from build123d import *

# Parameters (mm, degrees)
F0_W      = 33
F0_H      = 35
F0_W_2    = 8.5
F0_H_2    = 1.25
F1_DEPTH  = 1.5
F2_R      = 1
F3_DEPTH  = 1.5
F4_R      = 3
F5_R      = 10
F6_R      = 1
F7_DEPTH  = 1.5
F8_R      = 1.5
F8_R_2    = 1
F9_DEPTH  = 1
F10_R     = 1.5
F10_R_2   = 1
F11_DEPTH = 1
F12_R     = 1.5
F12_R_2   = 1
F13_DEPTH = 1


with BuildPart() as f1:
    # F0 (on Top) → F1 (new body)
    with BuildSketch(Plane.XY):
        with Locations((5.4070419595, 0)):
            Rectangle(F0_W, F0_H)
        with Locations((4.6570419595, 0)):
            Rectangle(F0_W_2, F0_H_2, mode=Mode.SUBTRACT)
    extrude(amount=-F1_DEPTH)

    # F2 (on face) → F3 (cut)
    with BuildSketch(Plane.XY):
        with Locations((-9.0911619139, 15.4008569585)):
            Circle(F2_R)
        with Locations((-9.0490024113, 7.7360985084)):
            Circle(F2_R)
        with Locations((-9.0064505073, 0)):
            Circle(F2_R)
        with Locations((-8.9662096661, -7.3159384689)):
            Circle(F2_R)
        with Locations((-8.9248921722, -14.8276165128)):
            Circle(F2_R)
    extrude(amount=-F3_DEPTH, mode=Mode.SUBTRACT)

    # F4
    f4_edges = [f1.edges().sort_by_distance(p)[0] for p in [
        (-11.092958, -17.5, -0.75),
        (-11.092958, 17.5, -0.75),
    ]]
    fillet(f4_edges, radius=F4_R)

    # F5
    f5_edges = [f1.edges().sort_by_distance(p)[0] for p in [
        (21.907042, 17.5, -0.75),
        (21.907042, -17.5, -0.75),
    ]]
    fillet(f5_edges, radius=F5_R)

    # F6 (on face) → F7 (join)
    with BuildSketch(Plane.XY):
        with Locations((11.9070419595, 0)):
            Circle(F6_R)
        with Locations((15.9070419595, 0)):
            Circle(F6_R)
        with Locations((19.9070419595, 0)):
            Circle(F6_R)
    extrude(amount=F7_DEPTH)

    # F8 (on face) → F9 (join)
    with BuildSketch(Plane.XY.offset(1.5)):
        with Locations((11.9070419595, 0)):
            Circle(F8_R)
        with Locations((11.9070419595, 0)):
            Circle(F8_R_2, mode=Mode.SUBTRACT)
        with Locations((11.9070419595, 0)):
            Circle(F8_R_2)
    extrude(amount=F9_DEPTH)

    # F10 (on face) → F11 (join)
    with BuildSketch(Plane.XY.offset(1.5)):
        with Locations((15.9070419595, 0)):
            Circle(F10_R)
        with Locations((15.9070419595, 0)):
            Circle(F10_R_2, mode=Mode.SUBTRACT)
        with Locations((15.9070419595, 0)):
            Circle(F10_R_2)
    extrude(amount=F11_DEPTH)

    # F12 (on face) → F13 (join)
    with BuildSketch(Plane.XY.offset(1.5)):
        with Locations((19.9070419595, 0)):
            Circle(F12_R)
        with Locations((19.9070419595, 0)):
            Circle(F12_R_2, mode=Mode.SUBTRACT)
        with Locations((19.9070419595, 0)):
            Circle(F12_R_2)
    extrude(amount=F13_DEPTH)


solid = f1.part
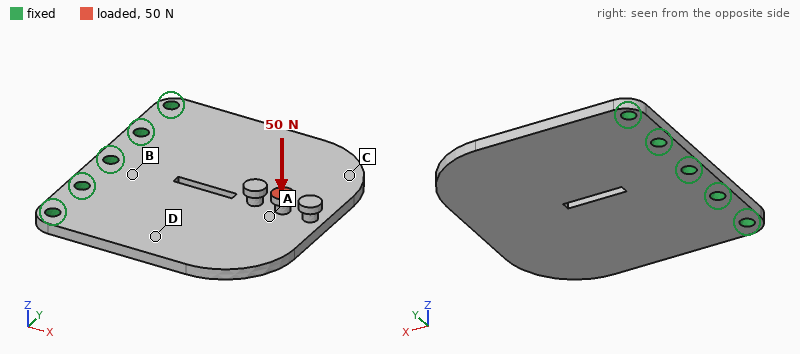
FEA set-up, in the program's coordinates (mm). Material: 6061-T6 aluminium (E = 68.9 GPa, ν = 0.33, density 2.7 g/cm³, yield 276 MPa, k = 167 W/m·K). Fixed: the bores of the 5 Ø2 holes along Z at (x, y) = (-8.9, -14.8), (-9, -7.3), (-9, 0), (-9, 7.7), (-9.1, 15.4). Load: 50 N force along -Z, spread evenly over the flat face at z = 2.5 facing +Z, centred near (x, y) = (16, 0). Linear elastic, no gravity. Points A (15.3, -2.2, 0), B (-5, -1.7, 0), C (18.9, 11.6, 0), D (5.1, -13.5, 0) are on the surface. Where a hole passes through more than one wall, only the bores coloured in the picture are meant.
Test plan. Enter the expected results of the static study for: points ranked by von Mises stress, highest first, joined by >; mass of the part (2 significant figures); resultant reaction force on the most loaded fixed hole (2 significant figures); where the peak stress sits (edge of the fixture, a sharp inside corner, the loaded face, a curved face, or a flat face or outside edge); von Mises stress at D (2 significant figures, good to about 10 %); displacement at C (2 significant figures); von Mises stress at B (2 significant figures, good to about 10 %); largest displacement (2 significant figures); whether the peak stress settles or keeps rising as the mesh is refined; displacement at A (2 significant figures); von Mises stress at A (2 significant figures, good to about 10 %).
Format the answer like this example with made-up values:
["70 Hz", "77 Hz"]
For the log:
["B > D > A > C", "4.5 g", "21 N", "edge of the fixture", "42 MPa", "0.41 mm", "76 MPa", "0.50 mm", "keeps rising", "0.35 mm", "23 MPa"]
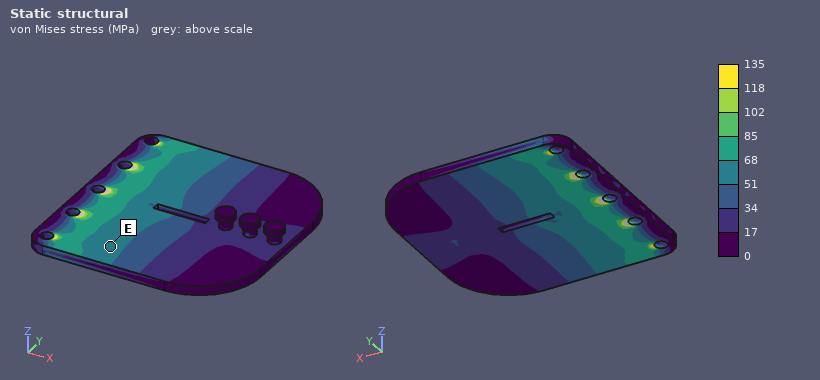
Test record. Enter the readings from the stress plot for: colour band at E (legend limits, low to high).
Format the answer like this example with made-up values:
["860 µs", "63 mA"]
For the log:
["51 to 68 MPa"]
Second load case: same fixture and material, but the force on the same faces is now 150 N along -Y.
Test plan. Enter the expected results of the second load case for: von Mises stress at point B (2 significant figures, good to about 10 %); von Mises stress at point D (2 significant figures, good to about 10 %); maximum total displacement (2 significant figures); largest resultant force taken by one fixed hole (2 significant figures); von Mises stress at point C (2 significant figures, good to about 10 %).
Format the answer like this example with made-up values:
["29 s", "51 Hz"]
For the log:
["19 MPa", "22 MPa", "0.12 mm", "110 N", "20 MPa"]
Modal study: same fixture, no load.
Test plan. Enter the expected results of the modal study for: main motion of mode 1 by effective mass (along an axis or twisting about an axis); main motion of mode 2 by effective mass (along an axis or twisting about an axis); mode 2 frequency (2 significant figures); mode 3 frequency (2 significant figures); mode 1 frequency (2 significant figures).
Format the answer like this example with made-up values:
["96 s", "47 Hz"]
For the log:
["along Z", "twisting about X", "3300 Hz", "7700 Hz", "1400 Hz"]
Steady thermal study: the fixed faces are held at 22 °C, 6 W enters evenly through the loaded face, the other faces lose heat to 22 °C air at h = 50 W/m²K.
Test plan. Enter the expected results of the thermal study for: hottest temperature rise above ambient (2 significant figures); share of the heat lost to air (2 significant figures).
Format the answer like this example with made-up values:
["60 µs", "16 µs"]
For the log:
["50 K", "18 %"]
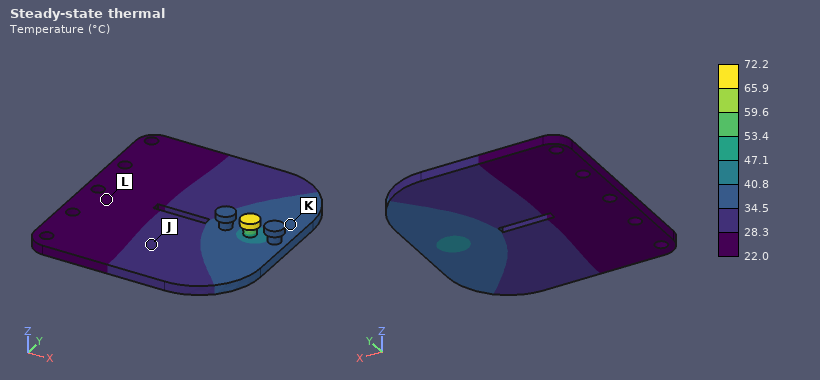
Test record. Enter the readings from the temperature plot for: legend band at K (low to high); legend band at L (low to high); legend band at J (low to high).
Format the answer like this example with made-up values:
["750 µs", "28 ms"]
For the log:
["34.5 to 40.8 °C", "22.0 to 28.3 °C", "28.3 to 34.5 °C"]
